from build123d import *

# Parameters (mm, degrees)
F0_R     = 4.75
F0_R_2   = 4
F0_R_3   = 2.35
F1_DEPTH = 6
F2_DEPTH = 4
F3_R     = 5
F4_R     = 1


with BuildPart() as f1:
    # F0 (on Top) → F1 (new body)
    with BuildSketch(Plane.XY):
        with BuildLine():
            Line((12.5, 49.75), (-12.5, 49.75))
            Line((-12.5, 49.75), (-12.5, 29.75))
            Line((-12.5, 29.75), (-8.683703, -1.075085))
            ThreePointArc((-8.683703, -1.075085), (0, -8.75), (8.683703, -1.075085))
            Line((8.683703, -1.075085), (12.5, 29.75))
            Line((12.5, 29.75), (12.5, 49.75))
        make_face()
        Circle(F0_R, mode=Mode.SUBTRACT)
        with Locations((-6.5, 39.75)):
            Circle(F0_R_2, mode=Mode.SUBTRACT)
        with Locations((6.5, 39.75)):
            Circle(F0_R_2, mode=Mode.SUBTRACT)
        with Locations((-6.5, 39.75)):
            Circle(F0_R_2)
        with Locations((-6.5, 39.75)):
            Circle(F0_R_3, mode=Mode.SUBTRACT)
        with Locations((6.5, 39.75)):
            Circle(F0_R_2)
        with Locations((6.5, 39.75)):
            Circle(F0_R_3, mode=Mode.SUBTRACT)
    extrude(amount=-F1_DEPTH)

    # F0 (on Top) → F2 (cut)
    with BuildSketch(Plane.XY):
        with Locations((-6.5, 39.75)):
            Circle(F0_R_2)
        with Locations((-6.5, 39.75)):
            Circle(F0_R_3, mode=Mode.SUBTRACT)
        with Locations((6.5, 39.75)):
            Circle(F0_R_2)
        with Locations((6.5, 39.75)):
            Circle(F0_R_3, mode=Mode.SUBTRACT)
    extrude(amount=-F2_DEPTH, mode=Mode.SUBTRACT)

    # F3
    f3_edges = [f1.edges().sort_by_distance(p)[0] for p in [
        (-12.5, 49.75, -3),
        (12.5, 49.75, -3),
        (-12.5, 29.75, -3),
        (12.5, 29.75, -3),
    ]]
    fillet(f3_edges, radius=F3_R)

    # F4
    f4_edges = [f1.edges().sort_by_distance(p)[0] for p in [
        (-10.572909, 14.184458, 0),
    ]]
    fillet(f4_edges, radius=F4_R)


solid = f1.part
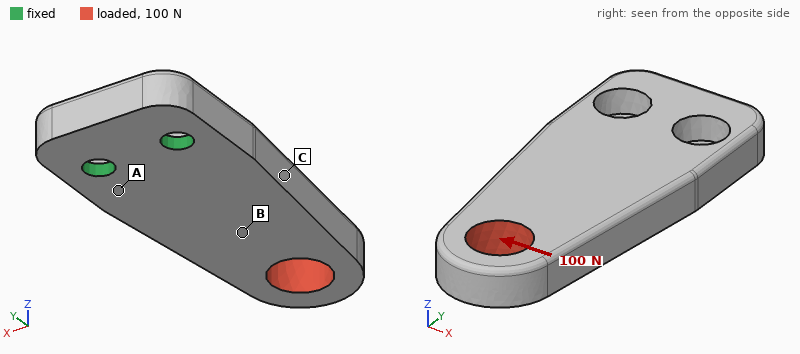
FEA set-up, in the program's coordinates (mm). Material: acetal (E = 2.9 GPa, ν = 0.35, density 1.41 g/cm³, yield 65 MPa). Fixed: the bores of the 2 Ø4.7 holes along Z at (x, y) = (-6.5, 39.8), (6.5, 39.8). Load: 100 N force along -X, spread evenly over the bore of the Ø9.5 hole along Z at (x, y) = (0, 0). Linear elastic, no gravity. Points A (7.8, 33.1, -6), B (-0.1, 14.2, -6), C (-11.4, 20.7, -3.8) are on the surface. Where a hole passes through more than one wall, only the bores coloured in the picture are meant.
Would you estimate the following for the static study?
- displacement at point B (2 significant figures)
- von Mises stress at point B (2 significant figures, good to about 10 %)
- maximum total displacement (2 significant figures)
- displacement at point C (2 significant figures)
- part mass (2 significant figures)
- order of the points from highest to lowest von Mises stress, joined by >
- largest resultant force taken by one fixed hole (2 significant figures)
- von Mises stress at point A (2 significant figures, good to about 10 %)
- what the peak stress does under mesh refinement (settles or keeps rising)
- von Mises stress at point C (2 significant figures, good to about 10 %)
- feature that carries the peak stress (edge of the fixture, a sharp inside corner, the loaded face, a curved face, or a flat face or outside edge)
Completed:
0.12 mm
2.1 MPa
0.29 mm
0.097 mm
9.2 g
A > C > B
250 N
7.5 MPa
keeps rising
4.4 MPa
edge of the fixture
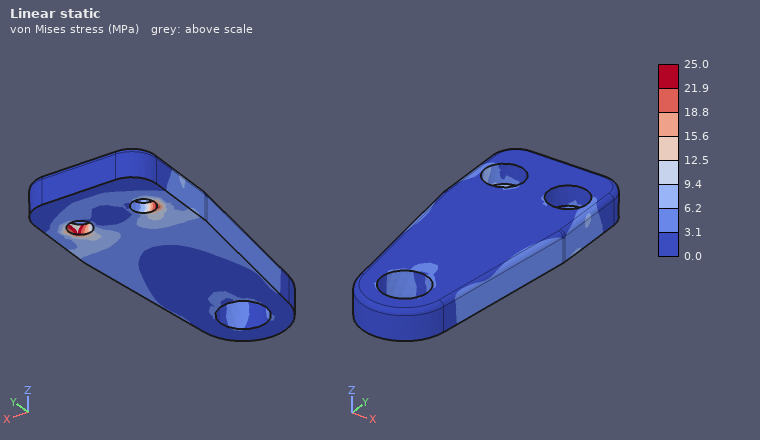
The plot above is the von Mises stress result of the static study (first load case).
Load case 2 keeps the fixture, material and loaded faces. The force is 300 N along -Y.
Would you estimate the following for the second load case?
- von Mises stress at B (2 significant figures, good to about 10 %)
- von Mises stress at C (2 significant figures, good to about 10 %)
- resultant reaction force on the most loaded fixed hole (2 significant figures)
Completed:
2.0 MPa
2.2 MPa
150 N
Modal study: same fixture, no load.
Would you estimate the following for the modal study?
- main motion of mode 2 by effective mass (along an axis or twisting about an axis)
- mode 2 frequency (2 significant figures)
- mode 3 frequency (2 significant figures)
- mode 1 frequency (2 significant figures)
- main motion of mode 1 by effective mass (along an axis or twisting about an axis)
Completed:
along X
2100 Hz
2900 Hz
570 Hz
along Z
